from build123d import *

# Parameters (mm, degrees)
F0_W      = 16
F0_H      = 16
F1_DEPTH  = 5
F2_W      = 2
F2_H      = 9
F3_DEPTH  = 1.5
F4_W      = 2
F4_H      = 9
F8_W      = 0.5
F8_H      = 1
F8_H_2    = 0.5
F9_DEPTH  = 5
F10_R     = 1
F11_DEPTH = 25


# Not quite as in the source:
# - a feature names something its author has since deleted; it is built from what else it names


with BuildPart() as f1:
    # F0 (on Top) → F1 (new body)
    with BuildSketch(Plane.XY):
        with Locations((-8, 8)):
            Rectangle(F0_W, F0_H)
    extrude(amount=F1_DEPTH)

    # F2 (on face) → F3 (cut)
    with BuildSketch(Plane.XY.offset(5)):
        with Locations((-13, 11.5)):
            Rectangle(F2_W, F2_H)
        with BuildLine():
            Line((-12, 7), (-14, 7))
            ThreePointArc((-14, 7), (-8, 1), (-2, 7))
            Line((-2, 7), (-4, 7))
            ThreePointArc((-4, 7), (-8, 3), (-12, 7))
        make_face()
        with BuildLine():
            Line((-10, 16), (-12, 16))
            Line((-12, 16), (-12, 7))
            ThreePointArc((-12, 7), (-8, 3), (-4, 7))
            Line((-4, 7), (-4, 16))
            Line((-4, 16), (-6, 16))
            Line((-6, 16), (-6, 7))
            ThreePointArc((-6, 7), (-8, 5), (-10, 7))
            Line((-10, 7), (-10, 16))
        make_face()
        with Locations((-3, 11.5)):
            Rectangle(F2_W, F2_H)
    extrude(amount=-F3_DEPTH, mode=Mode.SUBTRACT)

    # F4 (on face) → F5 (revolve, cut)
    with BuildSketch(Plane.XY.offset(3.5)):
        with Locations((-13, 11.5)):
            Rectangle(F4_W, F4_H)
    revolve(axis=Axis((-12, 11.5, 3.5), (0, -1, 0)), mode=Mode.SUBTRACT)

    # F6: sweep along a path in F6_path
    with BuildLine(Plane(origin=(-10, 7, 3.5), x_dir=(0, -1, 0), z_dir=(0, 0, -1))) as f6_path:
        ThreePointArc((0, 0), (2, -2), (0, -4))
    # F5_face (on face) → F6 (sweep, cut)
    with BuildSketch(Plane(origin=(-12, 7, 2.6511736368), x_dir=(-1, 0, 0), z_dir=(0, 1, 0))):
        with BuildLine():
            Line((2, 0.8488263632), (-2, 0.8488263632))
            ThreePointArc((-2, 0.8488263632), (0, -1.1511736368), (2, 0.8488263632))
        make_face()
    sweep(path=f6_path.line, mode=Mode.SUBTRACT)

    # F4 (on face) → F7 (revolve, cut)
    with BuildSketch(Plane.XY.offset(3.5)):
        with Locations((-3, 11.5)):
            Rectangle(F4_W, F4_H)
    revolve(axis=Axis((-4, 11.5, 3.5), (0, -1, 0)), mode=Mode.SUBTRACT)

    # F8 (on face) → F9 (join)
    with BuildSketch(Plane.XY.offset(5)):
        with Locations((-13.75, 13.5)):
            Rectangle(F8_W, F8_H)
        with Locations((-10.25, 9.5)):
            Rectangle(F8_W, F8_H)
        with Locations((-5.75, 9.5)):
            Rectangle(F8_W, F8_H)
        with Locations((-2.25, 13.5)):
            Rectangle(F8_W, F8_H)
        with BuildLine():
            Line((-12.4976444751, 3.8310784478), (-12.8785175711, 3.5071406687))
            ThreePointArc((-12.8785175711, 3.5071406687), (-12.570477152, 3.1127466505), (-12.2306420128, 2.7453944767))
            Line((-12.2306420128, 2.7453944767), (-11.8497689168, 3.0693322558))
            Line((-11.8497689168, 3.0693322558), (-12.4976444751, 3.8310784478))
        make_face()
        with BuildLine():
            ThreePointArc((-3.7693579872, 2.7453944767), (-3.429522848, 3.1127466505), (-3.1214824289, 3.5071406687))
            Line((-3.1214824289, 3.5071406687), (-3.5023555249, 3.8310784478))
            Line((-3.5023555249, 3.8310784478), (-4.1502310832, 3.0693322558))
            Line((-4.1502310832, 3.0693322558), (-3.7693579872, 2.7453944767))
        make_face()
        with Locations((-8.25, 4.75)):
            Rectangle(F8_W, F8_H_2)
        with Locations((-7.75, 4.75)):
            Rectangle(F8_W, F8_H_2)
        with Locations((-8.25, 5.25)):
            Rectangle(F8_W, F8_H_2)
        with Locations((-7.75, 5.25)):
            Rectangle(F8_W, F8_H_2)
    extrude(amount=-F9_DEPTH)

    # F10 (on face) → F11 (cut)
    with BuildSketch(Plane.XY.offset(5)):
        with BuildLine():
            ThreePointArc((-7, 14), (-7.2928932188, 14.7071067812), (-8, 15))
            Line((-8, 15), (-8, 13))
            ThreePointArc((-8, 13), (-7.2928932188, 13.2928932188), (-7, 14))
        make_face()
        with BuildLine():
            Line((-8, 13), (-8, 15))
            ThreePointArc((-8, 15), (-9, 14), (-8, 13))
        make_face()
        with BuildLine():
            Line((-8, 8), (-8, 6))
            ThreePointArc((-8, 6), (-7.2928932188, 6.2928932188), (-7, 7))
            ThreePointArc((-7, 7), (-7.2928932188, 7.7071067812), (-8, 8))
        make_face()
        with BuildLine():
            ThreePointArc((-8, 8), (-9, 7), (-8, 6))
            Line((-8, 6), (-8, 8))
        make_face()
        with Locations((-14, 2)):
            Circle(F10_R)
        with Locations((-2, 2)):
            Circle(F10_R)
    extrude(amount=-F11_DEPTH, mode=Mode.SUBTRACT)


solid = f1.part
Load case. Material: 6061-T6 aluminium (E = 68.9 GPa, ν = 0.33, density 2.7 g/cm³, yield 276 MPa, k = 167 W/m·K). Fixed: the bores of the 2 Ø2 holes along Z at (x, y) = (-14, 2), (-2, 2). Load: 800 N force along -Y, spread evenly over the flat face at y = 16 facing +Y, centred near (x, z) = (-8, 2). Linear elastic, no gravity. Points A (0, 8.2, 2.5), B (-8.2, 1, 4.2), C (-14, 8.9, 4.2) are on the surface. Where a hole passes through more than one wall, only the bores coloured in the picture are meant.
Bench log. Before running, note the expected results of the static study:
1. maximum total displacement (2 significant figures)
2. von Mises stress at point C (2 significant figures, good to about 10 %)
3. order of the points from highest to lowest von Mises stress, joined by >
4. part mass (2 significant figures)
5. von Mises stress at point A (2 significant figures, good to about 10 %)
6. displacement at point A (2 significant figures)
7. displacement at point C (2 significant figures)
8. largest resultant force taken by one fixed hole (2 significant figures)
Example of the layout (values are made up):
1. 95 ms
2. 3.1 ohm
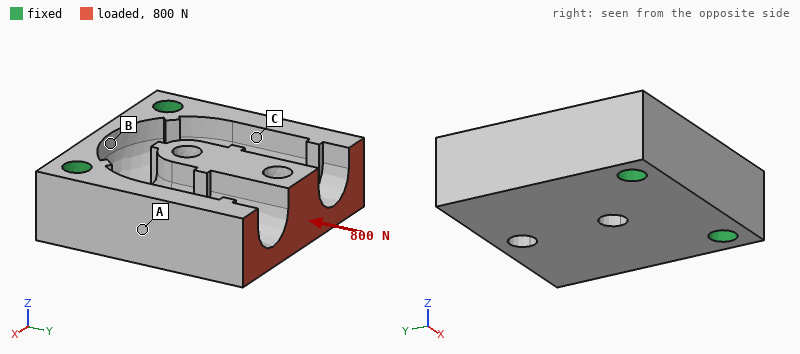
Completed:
1. 11 µm
2. 25 MPa
3. C > A > B
4. 2.3 g
5. 17 MPa
6. 2.1 µm
7. 2.7 µm
8. 400 N
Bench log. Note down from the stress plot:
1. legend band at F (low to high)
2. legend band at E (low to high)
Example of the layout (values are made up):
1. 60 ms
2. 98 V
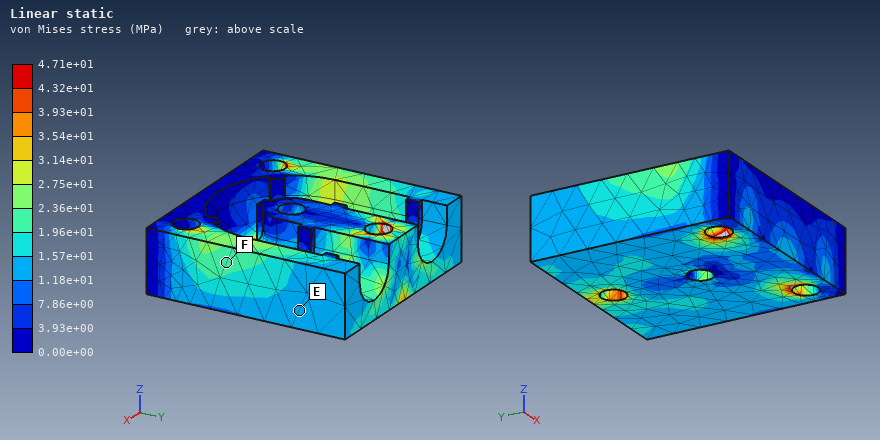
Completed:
1. 1.96e+01 to 2.36e+01 MPa
2. 1.18e+01 to 1.57e+01 MPa
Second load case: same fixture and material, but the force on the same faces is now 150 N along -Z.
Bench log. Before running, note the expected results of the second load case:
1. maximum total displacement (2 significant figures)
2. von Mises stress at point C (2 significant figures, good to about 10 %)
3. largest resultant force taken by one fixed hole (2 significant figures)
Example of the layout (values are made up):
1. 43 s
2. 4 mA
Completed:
1. 36 µm
2. 40 MPa
3. 76 N
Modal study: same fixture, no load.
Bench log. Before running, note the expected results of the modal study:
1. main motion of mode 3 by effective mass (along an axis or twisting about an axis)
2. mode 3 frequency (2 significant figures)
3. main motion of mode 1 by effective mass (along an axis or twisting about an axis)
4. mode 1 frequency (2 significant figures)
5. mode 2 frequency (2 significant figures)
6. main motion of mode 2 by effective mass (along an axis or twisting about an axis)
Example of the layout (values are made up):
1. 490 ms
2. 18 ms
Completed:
1. along X
2. 37 kHz
3. along Z
4. 15 kHz
5. 24 kHz
6. along X
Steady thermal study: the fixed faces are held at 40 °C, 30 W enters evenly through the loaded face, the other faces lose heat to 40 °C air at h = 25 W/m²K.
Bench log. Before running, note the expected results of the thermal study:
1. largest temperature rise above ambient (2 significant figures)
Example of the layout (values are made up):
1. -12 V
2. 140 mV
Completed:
1. 57 K
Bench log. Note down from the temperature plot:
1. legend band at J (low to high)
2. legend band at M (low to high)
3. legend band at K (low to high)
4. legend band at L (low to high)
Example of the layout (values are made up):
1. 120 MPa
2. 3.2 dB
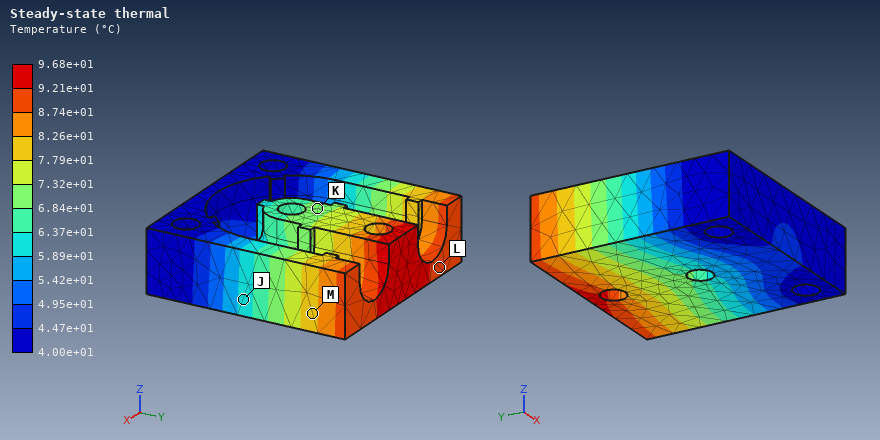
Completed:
1. 5.89e+01 to 6.37e+01 °C
2. 7.79e+01 to 8.26e+01 °C
3. 6.84e+01 to 7.32e+01 °C
4. 8.74e+01 to 9.21e+01 °C
